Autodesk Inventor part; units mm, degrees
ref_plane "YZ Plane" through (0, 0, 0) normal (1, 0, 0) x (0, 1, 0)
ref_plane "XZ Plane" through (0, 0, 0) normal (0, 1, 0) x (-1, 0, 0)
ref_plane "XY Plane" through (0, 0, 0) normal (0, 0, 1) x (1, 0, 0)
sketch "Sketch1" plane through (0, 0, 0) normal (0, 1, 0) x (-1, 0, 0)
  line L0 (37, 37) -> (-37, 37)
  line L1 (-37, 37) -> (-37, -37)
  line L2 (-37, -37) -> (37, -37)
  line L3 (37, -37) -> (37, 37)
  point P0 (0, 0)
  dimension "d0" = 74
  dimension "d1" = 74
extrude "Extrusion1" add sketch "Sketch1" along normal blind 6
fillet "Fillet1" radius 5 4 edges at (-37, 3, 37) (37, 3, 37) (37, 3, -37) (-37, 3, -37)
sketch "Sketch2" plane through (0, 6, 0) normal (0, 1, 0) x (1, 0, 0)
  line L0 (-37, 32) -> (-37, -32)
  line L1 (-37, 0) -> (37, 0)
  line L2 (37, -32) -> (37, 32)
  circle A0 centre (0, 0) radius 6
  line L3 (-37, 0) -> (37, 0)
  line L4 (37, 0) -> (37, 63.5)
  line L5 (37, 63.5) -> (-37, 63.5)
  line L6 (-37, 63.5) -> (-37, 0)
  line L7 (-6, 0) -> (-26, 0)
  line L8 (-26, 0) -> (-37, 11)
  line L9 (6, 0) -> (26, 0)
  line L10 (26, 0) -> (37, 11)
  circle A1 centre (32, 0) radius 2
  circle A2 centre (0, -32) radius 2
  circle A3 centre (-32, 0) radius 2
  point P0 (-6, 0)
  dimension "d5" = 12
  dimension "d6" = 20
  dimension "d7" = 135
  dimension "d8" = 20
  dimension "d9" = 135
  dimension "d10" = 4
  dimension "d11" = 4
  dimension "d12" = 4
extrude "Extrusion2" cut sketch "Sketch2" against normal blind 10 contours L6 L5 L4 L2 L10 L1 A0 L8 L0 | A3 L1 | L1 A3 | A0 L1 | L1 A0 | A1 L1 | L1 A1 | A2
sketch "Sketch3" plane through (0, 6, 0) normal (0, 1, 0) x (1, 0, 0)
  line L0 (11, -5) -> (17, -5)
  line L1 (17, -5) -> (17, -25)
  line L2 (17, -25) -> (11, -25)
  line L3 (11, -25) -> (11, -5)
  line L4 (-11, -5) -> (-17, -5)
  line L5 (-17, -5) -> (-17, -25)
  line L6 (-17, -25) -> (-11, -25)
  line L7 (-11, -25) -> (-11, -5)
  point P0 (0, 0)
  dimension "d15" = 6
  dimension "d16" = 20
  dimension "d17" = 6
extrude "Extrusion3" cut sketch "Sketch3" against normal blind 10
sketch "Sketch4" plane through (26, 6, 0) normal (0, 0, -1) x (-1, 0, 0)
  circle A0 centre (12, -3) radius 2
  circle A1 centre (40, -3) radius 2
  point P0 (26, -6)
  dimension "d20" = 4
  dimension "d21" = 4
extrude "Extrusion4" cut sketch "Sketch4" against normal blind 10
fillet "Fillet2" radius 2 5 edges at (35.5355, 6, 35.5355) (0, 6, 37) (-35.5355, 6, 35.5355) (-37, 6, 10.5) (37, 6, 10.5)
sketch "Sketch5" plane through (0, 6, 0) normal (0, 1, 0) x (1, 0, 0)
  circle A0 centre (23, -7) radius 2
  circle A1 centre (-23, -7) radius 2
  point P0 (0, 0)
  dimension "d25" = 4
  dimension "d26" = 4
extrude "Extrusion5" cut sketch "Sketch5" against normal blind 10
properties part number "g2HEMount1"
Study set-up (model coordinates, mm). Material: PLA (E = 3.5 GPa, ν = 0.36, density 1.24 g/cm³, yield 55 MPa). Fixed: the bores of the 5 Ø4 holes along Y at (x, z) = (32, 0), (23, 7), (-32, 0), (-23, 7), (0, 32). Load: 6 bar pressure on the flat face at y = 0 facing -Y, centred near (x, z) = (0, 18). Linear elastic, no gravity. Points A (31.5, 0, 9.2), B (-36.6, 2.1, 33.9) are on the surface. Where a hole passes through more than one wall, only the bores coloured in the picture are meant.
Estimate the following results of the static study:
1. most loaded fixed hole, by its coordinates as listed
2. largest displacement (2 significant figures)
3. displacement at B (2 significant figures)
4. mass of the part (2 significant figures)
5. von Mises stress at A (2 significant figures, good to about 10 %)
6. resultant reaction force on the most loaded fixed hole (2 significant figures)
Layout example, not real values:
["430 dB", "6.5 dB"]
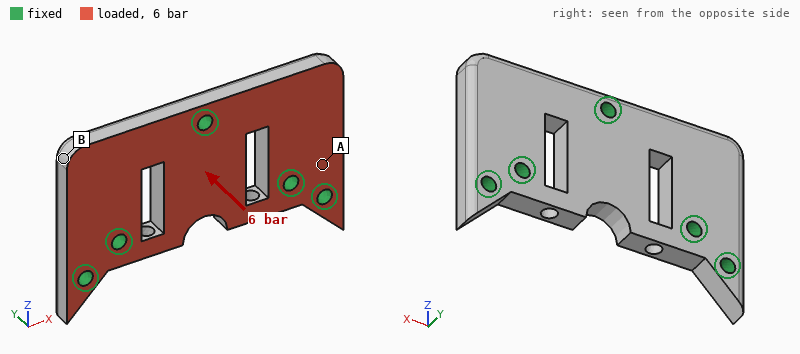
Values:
["(0, 32)", "0.57 mm", "0.55 mm", "18 g", "14 MPa", "570 N"]
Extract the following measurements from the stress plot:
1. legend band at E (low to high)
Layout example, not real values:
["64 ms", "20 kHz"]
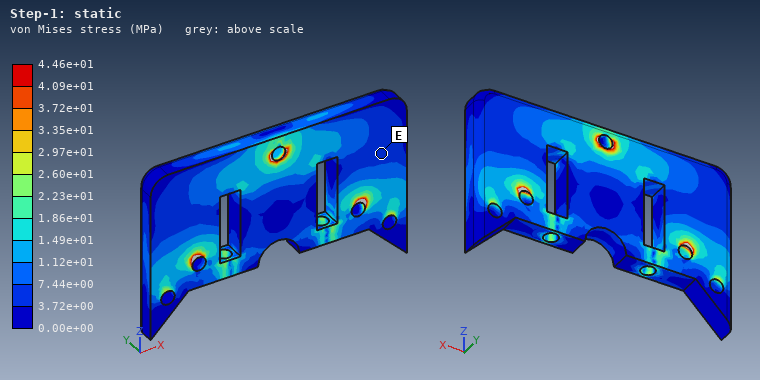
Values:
["3.72e+00 to 7.44e+00 MPa"]
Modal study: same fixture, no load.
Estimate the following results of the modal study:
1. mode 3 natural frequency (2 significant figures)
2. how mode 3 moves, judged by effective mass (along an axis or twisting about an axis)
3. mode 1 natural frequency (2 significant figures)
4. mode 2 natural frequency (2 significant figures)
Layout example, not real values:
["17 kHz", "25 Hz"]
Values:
["3900 Hz", "along Y", "2500 Hz", "2600 Hz"]
